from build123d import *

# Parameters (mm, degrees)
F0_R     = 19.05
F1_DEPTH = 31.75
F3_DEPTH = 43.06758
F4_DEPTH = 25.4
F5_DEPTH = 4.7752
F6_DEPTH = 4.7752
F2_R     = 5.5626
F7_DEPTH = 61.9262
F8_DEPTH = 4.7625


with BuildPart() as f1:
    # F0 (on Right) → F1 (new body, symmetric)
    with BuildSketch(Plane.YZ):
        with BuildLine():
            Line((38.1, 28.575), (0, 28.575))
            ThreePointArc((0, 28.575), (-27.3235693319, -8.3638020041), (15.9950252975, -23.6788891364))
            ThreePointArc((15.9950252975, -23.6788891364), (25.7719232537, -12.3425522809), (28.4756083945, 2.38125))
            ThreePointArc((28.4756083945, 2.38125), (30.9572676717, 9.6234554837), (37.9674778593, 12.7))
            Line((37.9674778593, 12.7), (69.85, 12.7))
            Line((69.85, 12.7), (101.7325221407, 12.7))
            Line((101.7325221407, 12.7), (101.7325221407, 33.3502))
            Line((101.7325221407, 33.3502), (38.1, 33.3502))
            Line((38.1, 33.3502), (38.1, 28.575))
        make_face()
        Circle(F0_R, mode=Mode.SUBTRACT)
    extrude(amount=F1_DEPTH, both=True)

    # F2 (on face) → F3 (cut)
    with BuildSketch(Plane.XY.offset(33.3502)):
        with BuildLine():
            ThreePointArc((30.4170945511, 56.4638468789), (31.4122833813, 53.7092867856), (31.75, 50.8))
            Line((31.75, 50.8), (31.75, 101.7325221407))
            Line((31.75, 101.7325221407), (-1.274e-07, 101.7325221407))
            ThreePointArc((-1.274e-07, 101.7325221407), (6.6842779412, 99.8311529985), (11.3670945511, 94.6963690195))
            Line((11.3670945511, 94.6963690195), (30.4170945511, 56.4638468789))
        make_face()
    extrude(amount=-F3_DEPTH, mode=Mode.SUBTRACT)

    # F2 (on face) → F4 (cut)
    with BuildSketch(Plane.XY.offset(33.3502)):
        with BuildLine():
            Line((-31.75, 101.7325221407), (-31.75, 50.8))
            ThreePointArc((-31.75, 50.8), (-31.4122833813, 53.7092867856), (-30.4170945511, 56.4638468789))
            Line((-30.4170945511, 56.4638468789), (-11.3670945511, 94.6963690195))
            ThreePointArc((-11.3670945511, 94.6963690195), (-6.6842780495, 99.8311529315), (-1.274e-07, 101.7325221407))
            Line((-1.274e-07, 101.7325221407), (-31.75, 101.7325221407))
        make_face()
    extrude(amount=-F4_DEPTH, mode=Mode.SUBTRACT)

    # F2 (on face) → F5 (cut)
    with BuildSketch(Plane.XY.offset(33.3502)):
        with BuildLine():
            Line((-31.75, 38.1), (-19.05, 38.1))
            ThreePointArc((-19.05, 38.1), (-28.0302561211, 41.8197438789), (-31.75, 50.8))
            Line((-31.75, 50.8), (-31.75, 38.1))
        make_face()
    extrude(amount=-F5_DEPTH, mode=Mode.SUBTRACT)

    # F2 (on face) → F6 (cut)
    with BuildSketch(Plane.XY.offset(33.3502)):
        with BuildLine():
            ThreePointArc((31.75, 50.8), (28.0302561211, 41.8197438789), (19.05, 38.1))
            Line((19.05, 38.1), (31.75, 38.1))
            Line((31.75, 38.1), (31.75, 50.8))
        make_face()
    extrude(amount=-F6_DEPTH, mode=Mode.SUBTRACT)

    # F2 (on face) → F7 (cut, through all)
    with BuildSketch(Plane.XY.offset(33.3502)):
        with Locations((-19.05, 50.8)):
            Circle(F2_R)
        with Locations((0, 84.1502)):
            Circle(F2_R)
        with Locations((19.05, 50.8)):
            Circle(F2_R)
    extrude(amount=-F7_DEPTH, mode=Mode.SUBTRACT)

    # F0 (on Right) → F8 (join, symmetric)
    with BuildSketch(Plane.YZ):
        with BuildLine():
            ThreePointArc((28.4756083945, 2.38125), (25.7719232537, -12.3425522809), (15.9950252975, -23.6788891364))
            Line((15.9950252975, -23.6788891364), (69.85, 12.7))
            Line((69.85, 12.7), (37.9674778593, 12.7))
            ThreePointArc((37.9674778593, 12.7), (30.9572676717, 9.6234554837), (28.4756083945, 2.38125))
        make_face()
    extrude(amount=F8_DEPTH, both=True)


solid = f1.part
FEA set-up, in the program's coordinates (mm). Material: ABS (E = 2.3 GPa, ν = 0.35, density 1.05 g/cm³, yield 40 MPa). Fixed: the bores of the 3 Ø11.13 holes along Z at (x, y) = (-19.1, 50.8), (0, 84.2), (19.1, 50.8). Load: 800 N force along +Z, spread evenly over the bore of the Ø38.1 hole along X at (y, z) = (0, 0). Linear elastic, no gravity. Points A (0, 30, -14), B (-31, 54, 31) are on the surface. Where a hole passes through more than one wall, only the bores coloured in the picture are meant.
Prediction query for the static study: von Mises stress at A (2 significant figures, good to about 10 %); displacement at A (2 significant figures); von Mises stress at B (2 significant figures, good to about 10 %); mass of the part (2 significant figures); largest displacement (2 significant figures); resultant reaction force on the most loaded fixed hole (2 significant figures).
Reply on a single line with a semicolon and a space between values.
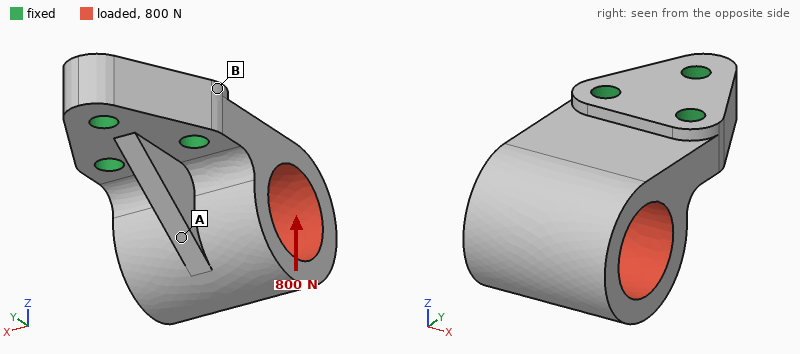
5.3 MPa; 0.25 mm; 1.2 MPa; 180 g; 0.66 mm; 560 N
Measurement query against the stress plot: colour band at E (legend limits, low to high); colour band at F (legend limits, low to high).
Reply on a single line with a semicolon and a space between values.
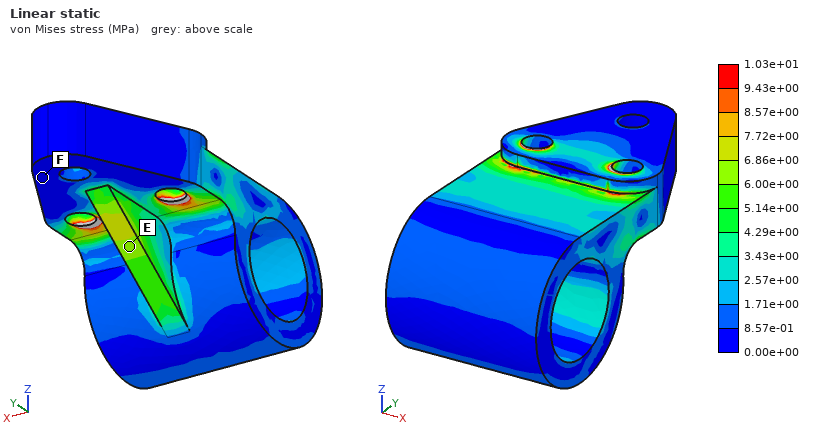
6.00e+00 to 6.86e+00 MPa; 0.00e+00 to 8.57e-01 MPa
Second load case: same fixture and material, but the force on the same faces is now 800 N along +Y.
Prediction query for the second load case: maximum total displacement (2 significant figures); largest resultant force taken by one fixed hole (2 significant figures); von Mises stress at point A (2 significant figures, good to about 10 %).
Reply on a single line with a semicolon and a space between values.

0.33 mm; 320 N; 4.5 MPa
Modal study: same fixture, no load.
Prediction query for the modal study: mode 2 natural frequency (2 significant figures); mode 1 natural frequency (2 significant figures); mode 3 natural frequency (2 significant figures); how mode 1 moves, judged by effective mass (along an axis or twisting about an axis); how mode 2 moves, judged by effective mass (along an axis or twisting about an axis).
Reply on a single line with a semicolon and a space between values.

1100 Hz; 600 Hz; 1800 Hz; along Z; along X
